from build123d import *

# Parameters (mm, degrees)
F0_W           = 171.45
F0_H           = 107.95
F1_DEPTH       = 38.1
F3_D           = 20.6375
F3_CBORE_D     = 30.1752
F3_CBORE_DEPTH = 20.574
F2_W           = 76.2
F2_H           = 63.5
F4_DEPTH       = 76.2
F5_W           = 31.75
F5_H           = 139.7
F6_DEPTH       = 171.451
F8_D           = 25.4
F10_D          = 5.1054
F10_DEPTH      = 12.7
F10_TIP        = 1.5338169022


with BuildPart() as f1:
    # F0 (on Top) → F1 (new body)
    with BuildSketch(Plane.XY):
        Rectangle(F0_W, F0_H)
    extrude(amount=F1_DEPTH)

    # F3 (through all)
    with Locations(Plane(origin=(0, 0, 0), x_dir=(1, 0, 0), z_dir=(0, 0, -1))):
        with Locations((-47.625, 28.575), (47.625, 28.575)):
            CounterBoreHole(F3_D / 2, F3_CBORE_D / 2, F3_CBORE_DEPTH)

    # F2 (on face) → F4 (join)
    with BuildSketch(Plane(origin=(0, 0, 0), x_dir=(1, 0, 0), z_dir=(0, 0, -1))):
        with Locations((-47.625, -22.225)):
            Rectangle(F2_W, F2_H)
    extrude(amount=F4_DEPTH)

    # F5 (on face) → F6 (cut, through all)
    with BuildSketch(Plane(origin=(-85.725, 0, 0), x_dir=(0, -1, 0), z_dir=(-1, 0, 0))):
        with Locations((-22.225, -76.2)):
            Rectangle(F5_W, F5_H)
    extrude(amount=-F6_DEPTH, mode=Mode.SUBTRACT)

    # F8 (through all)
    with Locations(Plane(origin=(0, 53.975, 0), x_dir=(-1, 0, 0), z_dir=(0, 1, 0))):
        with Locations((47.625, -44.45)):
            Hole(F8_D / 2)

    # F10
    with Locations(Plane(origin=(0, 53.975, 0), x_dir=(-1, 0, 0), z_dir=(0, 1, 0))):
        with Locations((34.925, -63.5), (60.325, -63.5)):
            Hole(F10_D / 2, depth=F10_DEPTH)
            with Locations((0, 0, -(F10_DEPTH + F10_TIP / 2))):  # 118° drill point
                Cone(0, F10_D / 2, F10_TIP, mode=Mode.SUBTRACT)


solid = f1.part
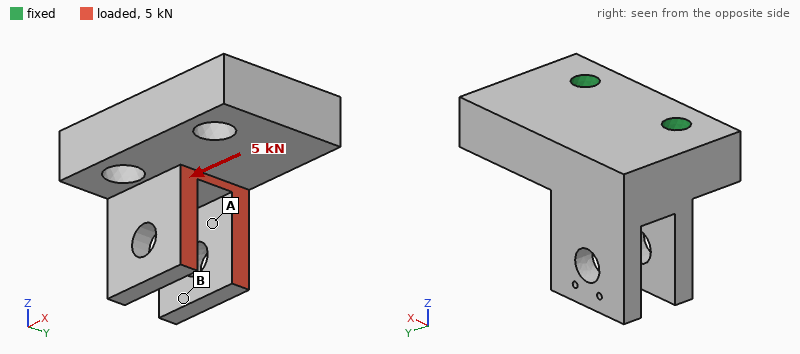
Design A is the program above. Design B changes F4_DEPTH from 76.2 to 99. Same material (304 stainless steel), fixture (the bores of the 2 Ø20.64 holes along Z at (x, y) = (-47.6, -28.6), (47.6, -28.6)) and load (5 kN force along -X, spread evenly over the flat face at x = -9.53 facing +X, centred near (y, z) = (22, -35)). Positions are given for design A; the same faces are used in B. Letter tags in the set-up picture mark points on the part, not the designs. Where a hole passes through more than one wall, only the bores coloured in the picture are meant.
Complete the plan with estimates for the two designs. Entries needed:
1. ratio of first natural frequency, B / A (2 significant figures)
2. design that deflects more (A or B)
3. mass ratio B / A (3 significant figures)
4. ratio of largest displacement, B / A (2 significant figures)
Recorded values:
0.72
B
1.07
1.5
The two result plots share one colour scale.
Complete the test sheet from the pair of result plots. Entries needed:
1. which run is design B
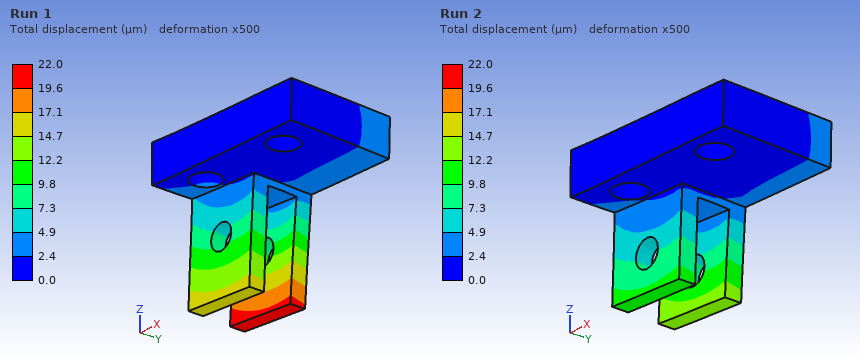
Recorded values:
Run 1
